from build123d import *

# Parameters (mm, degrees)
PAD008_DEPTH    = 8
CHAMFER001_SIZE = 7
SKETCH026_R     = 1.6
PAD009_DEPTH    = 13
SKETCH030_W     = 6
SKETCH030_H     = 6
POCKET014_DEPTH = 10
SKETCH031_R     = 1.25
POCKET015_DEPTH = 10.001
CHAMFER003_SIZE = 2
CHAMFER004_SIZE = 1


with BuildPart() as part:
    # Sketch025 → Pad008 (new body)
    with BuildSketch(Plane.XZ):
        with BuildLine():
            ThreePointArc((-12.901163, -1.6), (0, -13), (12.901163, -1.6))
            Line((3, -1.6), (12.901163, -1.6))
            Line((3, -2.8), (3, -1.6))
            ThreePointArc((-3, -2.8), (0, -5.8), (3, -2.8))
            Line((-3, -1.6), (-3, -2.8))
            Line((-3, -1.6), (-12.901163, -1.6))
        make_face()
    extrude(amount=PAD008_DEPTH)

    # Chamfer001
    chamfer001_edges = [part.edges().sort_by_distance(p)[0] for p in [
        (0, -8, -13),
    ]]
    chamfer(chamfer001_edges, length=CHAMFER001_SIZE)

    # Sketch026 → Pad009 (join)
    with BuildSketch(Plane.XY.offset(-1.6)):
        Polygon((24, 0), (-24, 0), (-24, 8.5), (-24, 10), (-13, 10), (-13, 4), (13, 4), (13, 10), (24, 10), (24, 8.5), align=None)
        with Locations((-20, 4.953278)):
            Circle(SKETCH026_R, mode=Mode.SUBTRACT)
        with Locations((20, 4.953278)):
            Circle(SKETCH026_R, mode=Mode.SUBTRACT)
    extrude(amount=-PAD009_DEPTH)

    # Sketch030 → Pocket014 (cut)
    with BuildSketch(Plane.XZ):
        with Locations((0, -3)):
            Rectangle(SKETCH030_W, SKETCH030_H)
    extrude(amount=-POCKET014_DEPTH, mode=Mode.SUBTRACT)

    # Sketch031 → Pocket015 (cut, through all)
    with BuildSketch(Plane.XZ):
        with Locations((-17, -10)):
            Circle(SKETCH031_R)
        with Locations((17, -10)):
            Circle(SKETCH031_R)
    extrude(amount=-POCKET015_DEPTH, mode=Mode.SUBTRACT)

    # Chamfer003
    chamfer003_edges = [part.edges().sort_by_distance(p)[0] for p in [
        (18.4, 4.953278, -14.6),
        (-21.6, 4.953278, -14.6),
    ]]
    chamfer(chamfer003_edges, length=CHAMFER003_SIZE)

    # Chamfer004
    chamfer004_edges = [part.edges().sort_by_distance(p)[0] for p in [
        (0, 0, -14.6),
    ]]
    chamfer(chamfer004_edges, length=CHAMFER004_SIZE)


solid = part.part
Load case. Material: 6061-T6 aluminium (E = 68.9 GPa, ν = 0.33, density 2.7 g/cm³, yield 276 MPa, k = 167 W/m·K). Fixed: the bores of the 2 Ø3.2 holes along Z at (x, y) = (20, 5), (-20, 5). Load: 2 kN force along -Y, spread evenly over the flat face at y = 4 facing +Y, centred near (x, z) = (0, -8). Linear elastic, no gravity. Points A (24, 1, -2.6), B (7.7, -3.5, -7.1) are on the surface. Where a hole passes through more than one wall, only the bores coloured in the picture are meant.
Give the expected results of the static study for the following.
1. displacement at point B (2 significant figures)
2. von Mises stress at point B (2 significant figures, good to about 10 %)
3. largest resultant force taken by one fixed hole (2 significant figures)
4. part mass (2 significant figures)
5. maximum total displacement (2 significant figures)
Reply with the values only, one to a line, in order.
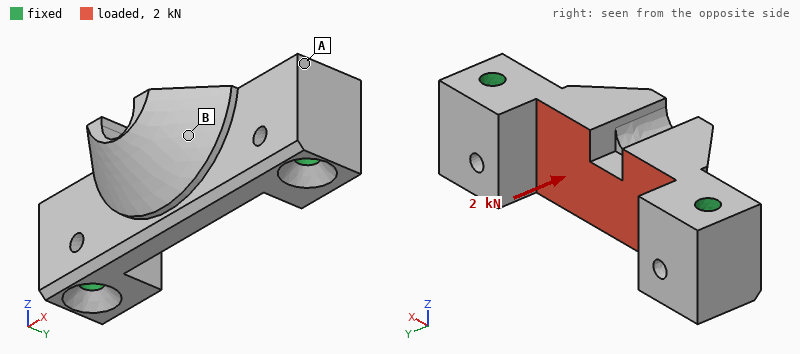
18 µm
41 MPa
1.3 kN
12 g
32 µm
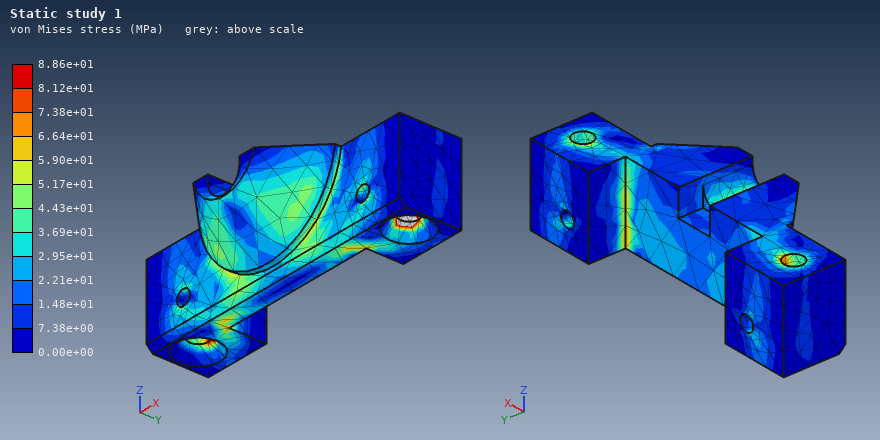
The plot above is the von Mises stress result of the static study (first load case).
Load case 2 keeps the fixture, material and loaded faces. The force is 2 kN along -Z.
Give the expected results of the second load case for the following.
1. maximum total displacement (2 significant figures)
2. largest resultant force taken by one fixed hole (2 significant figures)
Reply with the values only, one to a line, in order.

26 µm
1.0 kN
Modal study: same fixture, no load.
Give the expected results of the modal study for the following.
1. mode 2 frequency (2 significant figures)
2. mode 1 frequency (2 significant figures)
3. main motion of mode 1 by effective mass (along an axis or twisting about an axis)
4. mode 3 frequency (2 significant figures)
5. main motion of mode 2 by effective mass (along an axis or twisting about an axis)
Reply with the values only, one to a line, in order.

22 kHz
19 kHz
along Z
30 kHz
along Y
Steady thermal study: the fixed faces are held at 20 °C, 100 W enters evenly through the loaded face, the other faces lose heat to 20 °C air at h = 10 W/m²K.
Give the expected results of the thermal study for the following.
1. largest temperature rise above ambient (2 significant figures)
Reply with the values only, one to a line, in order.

60 K
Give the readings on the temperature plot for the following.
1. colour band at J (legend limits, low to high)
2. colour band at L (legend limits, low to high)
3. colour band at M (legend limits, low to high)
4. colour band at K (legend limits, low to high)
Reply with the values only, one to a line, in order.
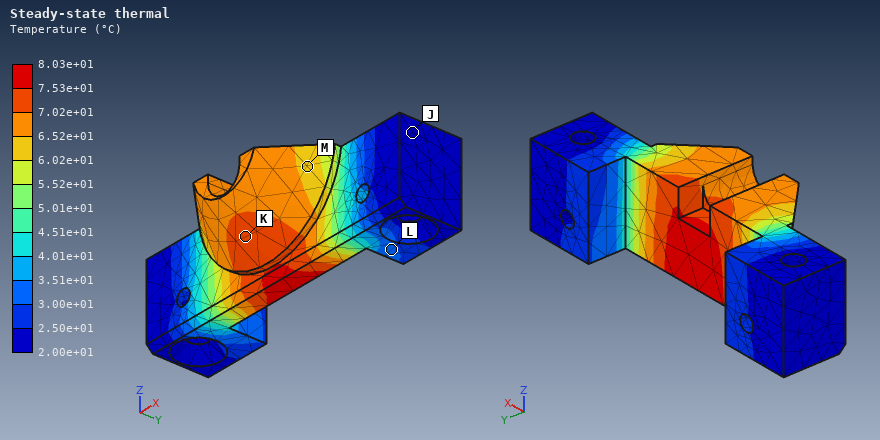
2.00e+01 to 2.50e+01 °C
3.00e+01 to 3.51e+01 °C
6.02e+01 to 6.52e+01 °C
7.02e+01 to 7.53e+01 °C
